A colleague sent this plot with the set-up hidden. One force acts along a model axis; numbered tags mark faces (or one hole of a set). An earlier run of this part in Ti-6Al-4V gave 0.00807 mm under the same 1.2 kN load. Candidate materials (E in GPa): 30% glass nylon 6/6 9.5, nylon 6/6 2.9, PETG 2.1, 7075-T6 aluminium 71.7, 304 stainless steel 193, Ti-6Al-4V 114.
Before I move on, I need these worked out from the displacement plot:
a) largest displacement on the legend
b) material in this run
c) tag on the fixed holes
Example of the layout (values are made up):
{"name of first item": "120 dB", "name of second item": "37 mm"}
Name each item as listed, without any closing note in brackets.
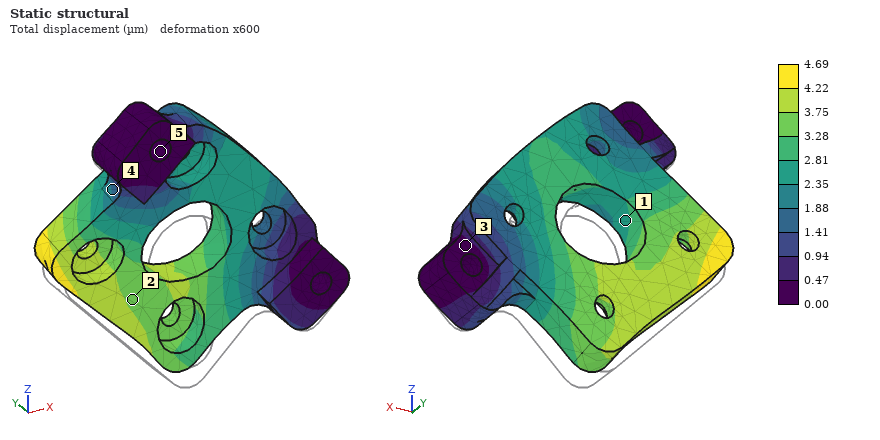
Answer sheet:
{"largest displacement on the legend": "4.69 µm", "material in this run": "304 stainless steel", "tag on the fixed holes": "5"}
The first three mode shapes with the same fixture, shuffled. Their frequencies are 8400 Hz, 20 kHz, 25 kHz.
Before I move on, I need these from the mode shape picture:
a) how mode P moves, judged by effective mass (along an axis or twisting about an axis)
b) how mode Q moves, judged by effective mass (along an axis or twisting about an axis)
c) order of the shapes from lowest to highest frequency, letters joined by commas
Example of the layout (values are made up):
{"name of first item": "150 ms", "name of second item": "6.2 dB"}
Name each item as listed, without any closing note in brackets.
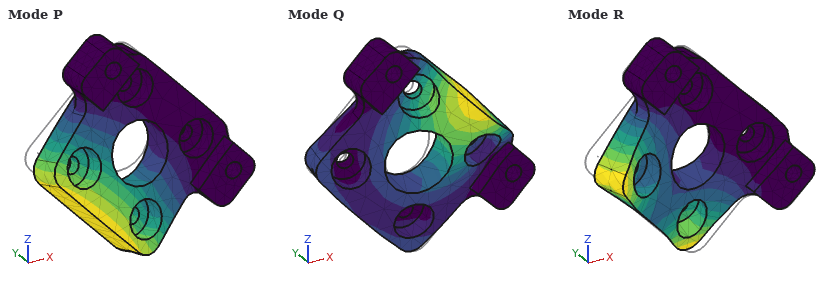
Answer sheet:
{"how mode P moves, judged by effective mass": "along Y", "how mode Q moves, judged by effective mass": "along Y", "order of the shapes from lowest to highest frequency, letters joined by commas": "P, R, Q"}
